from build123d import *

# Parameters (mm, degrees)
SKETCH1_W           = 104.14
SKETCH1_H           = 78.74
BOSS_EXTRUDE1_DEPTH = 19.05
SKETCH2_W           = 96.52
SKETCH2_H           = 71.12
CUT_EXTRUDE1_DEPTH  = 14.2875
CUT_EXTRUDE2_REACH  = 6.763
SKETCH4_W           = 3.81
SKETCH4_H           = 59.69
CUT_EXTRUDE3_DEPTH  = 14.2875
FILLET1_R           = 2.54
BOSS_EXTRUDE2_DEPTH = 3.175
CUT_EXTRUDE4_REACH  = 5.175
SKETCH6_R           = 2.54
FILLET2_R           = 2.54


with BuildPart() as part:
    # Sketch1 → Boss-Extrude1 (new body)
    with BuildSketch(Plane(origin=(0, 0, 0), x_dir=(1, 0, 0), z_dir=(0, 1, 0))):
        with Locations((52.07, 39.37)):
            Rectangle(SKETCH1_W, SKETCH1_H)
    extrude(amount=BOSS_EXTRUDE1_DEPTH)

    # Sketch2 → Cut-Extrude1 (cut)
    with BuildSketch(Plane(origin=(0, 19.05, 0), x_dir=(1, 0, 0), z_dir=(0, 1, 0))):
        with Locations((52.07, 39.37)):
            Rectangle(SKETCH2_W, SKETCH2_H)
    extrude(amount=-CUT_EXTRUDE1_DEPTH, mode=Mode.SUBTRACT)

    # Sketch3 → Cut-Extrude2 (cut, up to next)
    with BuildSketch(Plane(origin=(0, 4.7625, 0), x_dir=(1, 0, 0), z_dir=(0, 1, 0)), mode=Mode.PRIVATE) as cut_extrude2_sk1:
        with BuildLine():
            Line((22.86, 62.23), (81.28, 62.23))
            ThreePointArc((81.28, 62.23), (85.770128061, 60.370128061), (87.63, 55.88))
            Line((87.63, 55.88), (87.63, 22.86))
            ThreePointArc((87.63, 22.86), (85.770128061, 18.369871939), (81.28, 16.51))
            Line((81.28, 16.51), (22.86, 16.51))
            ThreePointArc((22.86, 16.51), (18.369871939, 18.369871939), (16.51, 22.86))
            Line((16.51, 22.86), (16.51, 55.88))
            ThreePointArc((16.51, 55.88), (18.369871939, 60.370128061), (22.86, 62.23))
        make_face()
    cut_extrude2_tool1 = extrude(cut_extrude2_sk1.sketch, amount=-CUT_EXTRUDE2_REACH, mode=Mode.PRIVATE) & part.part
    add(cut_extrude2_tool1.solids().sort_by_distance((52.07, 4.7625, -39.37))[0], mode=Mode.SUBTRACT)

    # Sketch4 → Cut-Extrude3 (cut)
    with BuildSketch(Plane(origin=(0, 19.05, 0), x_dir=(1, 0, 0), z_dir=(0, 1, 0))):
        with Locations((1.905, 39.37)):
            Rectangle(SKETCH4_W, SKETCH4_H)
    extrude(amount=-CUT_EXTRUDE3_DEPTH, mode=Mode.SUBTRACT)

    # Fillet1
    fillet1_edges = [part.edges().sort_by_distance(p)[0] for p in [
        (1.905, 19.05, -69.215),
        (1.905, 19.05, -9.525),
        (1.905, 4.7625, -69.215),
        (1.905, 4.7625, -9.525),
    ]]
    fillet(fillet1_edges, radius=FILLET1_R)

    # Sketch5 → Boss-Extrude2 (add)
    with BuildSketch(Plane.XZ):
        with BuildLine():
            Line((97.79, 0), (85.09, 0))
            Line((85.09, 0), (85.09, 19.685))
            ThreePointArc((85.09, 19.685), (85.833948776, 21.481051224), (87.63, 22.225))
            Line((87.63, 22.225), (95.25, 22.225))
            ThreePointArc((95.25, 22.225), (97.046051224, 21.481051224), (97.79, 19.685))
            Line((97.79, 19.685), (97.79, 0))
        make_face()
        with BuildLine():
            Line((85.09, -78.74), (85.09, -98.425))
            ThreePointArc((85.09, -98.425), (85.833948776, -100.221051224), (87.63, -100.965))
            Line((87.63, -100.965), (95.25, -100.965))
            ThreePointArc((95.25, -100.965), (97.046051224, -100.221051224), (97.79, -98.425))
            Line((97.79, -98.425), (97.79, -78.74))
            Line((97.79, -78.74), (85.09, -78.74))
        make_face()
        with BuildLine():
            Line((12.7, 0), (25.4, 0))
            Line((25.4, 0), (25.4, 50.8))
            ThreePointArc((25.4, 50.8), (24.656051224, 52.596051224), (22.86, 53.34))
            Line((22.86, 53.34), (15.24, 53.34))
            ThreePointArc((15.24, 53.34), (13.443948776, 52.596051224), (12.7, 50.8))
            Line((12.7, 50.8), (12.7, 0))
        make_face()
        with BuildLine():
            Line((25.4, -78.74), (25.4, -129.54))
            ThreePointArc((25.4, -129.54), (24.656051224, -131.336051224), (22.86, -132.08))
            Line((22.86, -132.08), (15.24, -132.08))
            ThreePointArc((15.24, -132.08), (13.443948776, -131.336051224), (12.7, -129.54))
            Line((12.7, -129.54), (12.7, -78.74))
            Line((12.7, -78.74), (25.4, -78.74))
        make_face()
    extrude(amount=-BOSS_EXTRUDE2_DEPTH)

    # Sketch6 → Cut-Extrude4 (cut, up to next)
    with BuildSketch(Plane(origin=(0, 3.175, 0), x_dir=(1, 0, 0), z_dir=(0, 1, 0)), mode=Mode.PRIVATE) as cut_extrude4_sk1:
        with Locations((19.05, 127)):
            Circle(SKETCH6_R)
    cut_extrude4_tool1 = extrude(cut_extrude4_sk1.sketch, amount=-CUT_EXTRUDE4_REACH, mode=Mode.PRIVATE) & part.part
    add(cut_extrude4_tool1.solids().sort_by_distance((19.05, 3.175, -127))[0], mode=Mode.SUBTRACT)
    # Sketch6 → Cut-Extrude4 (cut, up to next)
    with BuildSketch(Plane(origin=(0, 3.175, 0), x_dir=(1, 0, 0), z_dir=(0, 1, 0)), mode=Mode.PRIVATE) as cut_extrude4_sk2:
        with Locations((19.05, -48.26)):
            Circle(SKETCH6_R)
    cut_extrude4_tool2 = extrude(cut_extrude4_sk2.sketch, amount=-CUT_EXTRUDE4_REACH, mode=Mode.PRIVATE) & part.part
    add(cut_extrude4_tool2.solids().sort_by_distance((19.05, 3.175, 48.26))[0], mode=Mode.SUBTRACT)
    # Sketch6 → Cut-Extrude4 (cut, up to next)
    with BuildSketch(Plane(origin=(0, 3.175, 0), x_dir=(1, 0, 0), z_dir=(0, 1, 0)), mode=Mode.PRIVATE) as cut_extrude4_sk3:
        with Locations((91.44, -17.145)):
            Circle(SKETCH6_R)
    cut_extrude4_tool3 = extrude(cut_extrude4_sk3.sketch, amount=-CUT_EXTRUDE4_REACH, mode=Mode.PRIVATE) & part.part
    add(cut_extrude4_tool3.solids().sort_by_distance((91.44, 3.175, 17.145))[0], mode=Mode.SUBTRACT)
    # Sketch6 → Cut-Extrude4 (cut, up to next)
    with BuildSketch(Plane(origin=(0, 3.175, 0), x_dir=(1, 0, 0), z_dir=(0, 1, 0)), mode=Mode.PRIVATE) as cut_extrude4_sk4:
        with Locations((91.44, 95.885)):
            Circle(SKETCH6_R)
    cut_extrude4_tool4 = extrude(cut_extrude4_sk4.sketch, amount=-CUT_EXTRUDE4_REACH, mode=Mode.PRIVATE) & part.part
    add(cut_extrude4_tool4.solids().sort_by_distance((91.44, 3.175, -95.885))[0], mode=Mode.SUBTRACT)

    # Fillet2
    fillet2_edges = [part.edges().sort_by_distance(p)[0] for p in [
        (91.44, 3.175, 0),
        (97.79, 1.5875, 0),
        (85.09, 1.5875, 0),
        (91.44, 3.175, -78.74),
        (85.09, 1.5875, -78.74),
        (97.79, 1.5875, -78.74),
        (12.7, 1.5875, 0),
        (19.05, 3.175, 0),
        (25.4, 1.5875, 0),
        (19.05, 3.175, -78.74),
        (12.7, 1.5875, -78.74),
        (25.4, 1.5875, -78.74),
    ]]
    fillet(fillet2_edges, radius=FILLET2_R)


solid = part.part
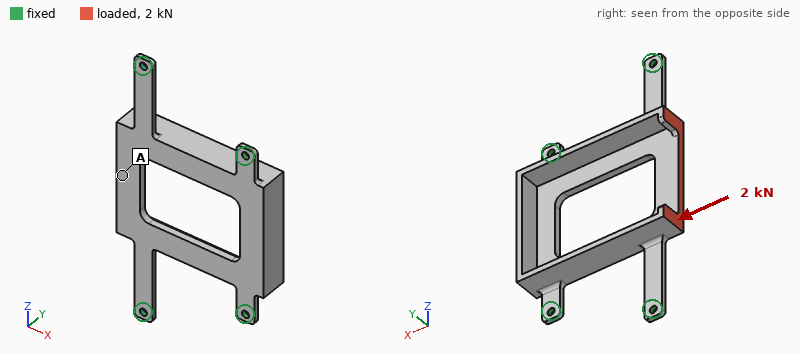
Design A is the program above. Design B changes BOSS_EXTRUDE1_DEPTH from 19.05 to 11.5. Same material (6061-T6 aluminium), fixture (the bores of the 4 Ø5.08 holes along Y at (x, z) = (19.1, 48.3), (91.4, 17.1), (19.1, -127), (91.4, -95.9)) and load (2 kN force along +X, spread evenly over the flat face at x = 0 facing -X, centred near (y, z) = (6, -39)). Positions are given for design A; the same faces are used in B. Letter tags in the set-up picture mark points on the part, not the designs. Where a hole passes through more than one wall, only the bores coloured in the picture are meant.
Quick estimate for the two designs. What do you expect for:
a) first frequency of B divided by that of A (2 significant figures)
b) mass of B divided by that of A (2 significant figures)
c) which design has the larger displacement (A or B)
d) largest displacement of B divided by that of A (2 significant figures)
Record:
1.1
0.82
A
0.50
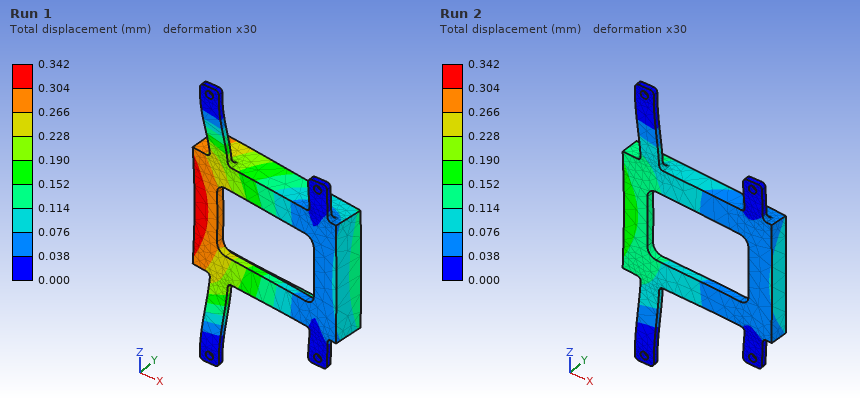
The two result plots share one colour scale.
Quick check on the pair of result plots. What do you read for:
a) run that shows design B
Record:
Run 2
